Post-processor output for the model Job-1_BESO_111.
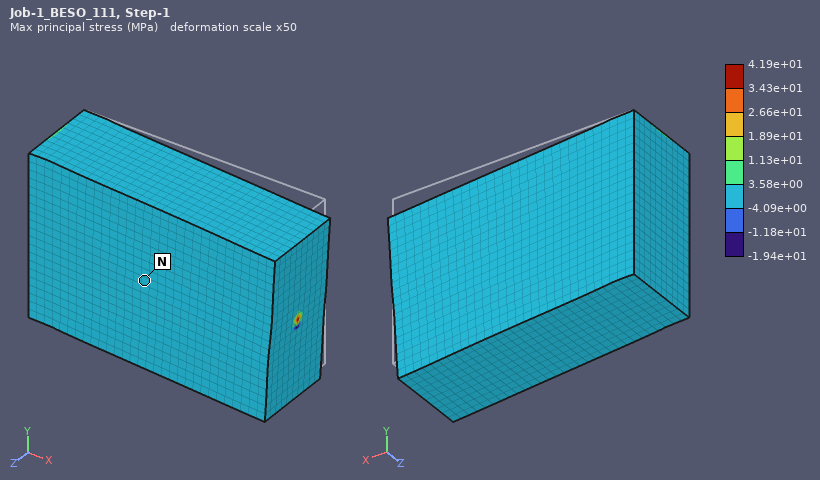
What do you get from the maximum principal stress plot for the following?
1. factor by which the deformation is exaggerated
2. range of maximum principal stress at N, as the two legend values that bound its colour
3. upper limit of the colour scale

50
-4.09e+00 to 3.58e+00 MPa
4.19e+01 MPa
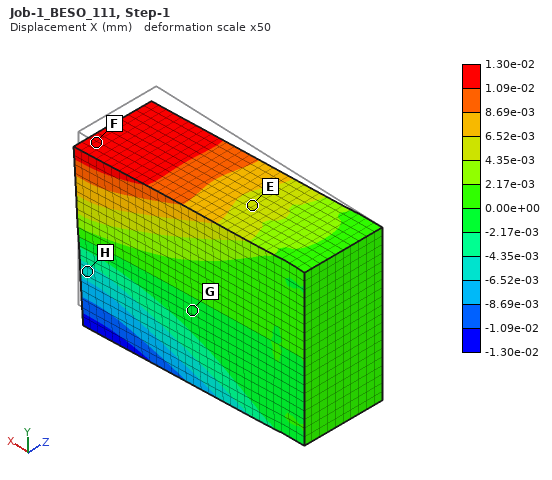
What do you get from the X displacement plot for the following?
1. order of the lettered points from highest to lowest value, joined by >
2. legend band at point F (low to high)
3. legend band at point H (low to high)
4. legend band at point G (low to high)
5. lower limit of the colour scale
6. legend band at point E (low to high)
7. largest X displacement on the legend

F > E > G > H
1.09e-02 to 1.30e-02 mm
-6.52e-03 to -4.35e-03 mm
-2.17e-03 to 0.00e+00 mm
-1.30e-02 mm
4.35e-03 to 6.52e-03 mm
1.30e-02 mm
